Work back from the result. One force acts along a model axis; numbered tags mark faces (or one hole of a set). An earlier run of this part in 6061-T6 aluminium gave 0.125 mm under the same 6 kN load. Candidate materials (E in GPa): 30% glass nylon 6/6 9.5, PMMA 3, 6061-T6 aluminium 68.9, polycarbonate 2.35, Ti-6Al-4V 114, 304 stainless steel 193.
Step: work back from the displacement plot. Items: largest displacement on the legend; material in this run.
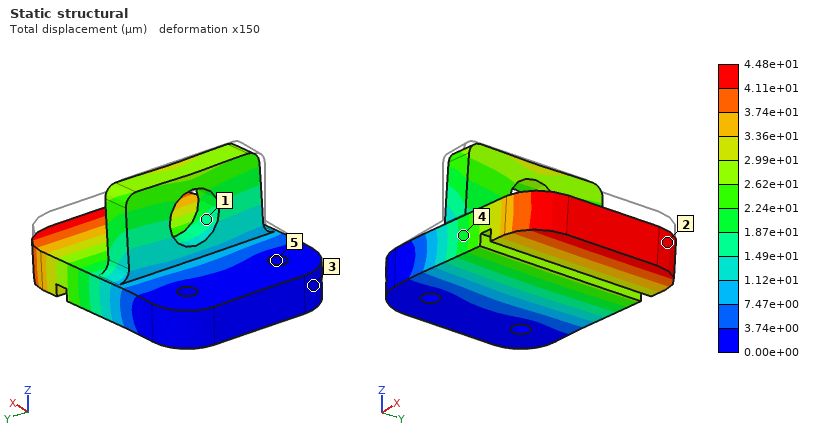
4.48e+01 µm
304 stainless steel
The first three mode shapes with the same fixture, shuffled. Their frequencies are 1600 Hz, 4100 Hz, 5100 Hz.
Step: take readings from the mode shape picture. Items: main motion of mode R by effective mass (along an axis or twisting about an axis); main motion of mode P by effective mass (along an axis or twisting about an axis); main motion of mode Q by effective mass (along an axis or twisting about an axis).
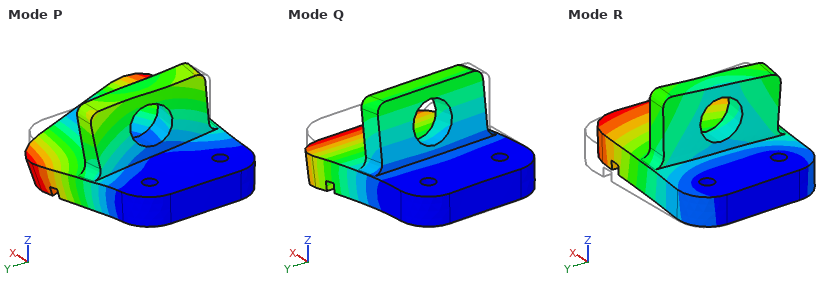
along Y
twisting about X
along Z
